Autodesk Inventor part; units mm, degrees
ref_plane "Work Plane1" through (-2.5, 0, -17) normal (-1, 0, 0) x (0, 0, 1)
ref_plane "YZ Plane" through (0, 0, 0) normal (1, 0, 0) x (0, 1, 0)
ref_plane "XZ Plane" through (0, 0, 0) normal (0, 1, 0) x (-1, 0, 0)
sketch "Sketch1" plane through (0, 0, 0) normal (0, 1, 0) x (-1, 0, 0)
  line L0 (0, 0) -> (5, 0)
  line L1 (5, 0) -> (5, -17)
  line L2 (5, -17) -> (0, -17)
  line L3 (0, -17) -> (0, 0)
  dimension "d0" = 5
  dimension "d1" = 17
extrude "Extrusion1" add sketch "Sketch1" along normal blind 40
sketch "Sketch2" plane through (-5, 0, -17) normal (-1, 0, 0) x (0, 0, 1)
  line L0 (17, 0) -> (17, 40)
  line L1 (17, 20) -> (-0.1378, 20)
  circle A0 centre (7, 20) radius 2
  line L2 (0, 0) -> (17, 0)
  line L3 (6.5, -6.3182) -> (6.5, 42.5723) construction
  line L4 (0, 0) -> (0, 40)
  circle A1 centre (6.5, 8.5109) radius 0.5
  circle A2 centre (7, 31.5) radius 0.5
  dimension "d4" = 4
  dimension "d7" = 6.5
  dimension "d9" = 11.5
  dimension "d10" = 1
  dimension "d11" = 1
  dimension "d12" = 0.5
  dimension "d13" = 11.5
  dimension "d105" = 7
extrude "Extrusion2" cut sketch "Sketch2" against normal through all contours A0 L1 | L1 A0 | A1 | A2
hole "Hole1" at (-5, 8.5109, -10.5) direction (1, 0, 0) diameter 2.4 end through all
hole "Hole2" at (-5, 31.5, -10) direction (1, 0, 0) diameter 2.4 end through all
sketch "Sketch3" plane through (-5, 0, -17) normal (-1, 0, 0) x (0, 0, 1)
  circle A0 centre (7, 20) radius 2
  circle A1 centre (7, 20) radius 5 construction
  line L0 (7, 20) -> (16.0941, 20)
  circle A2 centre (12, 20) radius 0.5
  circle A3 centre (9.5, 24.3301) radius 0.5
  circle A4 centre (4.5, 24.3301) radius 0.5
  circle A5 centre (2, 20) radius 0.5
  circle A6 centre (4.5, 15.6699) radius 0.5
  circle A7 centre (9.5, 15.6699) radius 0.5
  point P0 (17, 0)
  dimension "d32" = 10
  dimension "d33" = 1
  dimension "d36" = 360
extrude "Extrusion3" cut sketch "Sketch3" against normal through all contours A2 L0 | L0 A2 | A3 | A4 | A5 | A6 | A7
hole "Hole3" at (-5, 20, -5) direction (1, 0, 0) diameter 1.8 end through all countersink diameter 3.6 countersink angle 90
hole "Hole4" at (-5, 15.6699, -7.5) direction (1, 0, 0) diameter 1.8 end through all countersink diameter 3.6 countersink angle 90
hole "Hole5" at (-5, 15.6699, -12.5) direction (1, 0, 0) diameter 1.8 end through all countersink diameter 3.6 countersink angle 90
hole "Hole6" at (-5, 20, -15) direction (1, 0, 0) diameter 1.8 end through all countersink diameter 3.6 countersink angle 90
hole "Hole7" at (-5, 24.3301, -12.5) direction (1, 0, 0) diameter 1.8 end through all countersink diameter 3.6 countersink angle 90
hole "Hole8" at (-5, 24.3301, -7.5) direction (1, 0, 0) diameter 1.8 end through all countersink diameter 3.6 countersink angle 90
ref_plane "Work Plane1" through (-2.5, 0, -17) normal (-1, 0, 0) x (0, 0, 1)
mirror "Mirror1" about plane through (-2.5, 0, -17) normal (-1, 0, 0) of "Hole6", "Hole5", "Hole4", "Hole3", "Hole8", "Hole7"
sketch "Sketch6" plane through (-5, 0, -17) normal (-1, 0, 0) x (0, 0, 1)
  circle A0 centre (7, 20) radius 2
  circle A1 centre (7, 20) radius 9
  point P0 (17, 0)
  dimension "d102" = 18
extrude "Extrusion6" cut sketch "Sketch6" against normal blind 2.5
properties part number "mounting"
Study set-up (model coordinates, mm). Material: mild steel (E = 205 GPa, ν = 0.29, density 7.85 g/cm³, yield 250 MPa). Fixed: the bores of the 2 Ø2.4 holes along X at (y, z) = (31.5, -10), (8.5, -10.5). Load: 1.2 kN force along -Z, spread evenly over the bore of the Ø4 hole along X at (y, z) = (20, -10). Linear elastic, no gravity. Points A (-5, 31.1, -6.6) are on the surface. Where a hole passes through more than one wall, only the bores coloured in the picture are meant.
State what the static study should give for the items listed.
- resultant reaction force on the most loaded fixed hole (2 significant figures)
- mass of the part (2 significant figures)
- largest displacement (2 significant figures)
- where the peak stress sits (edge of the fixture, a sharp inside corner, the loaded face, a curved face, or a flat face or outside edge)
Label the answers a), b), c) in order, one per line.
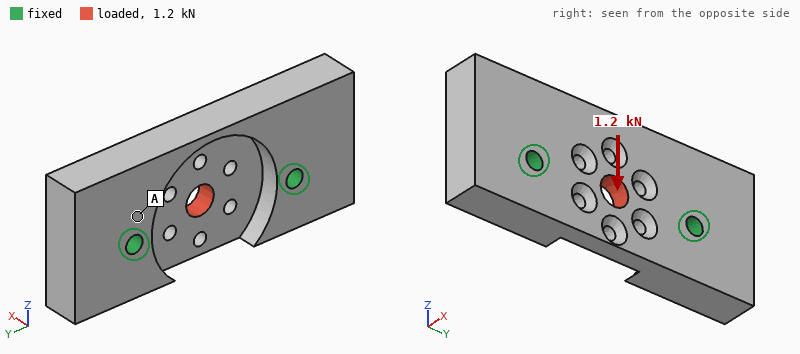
a) 630 N
b) 21 g
c) 4.2 µm
d) a curved face
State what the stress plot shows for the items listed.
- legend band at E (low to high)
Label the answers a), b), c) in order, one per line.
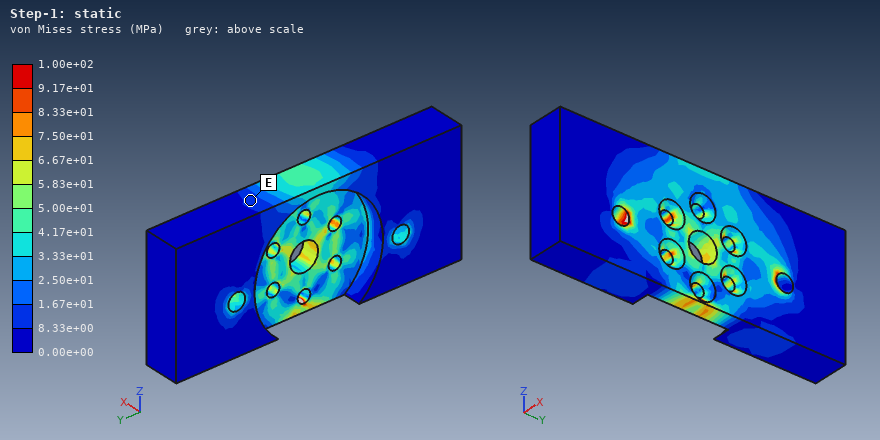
a) 8.33e+00 to 1.67e+01 MPa
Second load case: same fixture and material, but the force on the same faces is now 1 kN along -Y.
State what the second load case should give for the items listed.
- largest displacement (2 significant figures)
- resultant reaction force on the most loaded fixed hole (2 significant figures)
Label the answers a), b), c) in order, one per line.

a) 1.4 µm
b) 510 N
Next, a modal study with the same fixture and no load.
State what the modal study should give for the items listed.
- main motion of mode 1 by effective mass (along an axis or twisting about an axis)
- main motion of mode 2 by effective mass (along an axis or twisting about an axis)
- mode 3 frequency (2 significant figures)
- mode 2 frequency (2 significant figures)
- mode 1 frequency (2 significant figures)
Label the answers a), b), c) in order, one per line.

a) along X
b) twisting about Z
c) 28 kHz
d) 27 kHz
e) 23 kHz
